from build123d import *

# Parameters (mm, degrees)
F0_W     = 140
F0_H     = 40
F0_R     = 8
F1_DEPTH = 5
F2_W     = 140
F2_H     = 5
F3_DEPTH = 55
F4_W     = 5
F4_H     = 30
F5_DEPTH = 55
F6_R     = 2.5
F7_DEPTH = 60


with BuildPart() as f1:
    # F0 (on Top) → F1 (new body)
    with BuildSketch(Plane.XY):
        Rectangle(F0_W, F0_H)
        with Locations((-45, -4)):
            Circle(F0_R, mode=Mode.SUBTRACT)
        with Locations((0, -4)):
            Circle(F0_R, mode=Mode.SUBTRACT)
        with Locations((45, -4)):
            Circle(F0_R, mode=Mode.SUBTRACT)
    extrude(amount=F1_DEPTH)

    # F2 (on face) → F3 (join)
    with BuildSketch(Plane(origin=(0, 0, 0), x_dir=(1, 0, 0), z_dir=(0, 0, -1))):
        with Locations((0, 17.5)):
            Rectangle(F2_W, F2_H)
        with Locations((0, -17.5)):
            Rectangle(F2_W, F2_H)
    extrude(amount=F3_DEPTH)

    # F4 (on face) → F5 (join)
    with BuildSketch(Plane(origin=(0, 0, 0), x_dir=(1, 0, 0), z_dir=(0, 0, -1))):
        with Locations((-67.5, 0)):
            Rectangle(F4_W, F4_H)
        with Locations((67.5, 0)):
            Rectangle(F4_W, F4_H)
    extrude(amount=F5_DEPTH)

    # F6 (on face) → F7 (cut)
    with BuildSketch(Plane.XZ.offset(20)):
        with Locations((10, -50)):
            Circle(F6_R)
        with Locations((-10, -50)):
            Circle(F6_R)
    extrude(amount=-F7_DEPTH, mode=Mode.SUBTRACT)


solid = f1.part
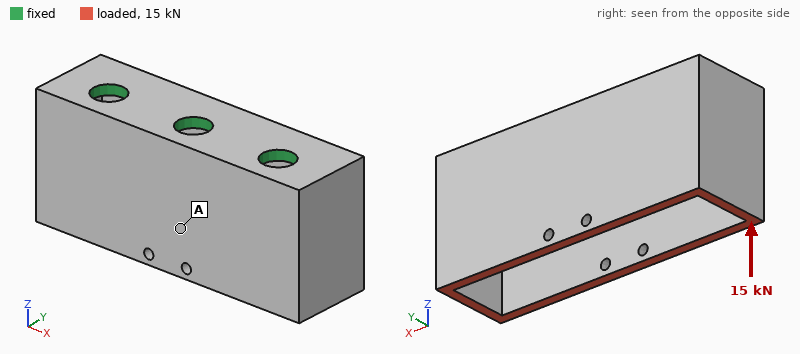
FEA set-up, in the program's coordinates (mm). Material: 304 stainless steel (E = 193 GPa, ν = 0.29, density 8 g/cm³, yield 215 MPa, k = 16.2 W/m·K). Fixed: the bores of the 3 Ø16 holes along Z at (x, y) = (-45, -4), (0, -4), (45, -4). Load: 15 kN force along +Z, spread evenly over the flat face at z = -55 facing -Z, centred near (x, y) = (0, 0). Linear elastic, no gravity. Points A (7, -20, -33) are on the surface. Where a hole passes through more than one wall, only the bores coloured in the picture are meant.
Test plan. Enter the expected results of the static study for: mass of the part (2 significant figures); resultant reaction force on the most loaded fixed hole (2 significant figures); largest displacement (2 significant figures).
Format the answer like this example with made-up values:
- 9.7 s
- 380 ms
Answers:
- 940 g
- 5.7 kN
- 83 µm
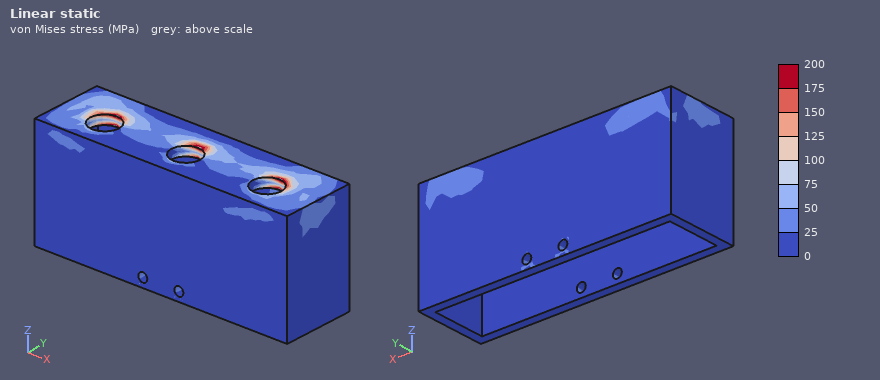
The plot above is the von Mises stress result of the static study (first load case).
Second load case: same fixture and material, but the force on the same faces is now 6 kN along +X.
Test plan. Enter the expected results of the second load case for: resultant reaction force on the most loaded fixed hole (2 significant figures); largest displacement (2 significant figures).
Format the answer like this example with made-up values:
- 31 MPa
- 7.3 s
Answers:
- 3.8 kN
- 37 µm
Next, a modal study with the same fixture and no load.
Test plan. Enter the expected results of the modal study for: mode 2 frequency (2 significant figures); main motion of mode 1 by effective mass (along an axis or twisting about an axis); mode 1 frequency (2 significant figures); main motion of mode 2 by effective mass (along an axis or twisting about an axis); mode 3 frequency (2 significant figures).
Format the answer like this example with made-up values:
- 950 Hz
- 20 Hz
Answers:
- 1800 Hz
- along Y
- 1400 Hz
- twisting about Z
- 1900 Hz
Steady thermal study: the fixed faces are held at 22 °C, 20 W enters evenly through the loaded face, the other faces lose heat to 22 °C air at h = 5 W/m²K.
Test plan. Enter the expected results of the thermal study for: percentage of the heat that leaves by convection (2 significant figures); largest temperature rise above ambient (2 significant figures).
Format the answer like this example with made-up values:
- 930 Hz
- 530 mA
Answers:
- 27 %
- 47 K
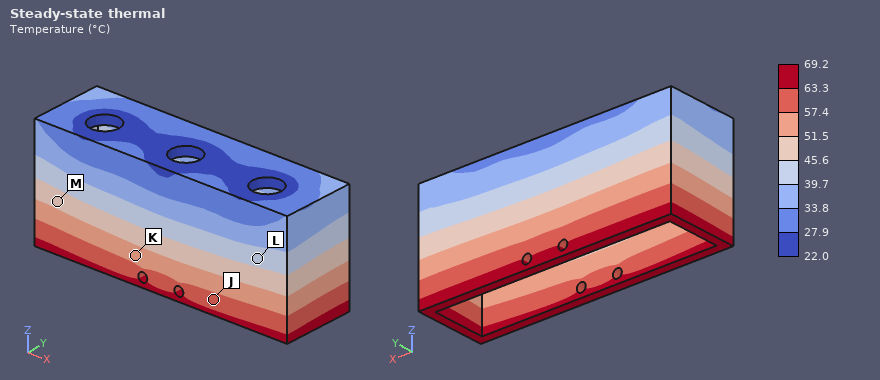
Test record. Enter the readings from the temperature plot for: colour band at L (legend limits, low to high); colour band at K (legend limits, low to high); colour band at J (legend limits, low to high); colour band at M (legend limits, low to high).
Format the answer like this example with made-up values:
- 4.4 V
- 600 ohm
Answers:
- 39.7 to 45.6 °C
- 51.5 to 57.4 °C
- 57.4 to 63.3 °C
- 45.6 to 51.5 °C
